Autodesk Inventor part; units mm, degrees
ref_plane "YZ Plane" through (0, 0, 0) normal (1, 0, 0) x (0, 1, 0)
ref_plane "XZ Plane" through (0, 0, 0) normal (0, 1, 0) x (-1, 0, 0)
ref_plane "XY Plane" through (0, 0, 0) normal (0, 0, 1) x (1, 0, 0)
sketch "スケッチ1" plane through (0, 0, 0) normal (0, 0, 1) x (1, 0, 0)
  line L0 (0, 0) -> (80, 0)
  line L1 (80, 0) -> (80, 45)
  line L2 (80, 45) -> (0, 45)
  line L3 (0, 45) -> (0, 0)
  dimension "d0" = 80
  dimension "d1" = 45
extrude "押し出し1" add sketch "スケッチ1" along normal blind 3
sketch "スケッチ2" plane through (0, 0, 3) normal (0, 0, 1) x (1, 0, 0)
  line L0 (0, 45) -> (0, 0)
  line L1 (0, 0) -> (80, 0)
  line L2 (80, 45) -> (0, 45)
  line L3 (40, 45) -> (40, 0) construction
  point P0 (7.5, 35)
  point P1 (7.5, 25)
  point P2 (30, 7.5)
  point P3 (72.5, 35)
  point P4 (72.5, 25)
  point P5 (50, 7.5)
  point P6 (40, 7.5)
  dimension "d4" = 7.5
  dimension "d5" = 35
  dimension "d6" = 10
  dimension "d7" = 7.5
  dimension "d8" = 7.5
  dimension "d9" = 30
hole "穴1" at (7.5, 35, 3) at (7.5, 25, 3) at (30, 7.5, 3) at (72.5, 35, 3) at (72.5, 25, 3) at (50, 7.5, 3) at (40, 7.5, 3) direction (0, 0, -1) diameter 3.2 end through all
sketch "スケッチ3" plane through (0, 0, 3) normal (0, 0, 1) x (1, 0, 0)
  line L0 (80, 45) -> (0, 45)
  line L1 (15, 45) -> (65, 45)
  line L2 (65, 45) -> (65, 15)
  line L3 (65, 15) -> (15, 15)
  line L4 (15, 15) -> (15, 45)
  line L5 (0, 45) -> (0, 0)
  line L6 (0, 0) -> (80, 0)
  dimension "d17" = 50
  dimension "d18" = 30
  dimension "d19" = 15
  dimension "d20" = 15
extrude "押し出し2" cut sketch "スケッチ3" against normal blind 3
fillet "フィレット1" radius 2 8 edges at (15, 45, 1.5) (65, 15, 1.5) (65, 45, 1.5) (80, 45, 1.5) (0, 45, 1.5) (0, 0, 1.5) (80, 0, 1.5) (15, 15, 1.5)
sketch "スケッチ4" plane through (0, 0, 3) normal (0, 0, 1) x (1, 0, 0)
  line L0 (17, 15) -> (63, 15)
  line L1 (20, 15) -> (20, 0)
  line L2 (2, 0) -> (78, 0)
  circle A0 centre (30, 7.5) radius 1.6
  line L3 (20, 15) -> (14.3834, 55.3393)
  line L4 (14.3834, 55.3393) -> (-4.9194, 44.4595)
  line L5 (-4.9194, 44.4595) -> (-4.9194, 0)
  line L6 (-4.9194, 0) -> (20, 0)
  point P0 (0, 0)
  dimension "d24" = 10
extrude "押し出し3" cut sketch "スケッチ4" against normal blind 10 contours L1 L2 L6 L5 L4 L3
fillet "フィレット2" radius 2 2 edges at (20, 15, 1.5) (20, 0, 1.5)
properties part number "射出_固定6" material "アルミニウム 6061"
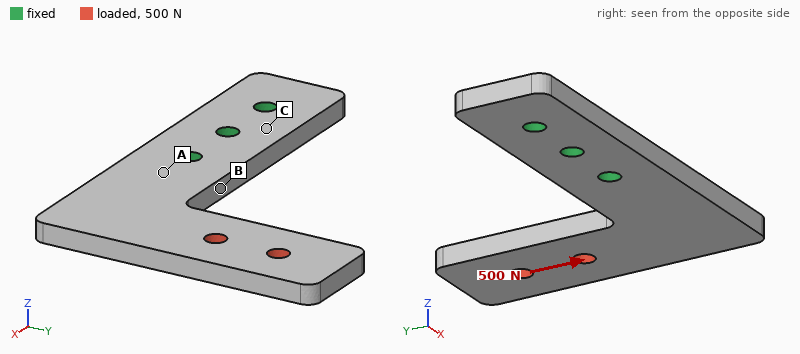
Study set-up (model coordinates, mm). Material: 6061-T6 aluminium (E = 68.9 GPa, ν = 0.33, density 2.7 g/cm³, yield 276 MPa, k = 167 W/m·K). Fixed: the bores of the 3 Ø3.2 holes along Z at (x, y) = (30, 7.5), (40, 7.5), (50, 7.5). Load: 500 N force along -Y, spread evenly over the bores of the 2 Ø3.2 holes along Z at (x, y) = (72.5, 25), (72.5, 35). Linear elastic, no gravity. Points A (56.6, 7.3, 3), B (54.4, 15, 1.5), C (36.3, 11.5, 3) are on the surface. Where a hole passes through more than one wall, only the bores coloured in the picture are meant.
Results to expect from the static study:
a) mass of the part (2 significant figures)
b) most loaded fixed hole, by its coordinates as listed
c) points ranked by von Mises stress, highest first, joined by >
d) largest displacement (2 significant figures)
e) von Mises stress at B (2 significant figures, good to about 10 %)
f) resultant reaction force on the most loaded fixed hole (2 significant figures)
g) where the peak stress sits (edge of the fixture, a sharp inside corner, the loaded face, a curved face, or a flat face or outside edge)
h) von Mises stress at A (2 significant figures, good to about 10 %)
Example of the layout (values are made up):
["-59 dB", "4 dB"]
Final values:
["11 g", "(50, 7.5)", "B > A > C", "0.16 mm", "85 MPa", "1.1 kN", "edge of the fixture", "29 MPa"]
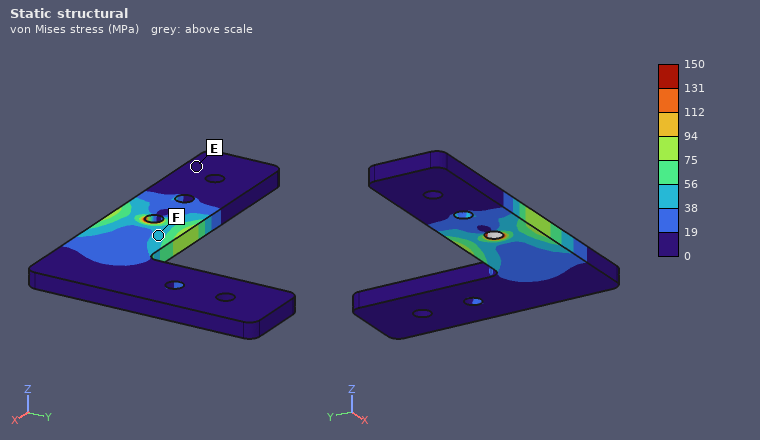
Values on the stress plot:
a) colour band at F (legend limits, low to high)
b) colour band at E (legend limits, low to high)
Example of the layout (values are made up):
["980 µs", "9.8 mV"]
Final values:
["38 to 56 MPa", "0 to 19 MPa"]
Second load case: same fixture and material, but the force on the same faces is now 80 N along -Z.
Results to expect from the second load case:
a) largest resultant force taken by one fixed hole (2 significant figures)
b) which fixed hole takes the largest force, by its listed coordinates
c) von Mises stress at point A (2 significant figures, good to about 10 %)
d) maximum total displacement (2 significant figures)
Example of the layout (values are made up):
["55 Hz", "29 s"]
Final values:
["130 N", "(50, 7.5)", "87 MPa", "0.75 mm"]
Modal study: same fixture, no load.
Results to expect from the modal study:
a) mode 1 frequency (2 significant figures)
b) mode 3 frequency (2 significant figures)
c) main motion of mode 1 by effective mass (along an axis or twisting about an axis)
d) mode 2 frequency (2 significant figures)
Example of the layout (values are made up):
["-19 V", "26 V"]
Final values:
["1100 Hz", "3800 Hz", "along Z", "2600 Hz"]
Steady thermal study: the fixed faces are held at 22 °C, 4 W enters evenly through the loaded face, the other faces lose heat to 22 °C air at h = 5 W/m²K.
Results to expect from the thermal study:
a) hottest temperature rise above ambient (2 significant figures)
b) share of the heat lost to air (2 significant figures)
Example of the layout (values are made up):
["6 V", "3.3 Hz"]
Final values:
["21 K", "3.4 %"]
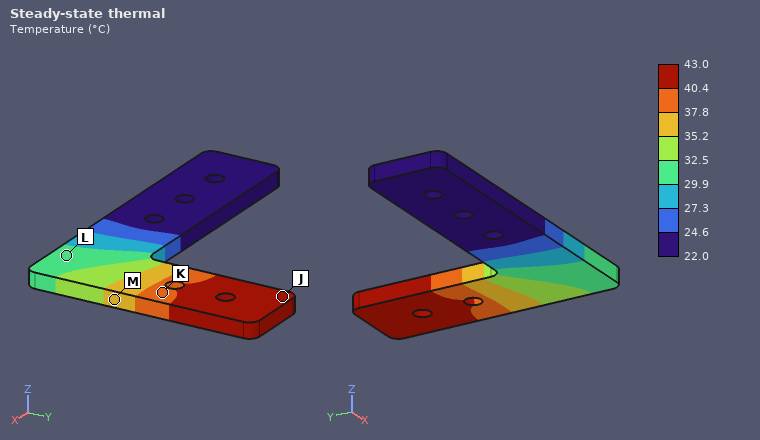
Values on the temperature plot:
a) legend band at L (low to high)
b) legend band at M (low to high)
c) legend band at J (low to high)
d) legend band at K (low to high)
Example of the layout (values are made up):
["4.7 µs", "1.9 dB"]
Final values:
["29.9 to 32.5 °C", "35.2 to 37.8 °C", "40.4 to 43.0 °C", "37.8 to 40.4 °C"]
